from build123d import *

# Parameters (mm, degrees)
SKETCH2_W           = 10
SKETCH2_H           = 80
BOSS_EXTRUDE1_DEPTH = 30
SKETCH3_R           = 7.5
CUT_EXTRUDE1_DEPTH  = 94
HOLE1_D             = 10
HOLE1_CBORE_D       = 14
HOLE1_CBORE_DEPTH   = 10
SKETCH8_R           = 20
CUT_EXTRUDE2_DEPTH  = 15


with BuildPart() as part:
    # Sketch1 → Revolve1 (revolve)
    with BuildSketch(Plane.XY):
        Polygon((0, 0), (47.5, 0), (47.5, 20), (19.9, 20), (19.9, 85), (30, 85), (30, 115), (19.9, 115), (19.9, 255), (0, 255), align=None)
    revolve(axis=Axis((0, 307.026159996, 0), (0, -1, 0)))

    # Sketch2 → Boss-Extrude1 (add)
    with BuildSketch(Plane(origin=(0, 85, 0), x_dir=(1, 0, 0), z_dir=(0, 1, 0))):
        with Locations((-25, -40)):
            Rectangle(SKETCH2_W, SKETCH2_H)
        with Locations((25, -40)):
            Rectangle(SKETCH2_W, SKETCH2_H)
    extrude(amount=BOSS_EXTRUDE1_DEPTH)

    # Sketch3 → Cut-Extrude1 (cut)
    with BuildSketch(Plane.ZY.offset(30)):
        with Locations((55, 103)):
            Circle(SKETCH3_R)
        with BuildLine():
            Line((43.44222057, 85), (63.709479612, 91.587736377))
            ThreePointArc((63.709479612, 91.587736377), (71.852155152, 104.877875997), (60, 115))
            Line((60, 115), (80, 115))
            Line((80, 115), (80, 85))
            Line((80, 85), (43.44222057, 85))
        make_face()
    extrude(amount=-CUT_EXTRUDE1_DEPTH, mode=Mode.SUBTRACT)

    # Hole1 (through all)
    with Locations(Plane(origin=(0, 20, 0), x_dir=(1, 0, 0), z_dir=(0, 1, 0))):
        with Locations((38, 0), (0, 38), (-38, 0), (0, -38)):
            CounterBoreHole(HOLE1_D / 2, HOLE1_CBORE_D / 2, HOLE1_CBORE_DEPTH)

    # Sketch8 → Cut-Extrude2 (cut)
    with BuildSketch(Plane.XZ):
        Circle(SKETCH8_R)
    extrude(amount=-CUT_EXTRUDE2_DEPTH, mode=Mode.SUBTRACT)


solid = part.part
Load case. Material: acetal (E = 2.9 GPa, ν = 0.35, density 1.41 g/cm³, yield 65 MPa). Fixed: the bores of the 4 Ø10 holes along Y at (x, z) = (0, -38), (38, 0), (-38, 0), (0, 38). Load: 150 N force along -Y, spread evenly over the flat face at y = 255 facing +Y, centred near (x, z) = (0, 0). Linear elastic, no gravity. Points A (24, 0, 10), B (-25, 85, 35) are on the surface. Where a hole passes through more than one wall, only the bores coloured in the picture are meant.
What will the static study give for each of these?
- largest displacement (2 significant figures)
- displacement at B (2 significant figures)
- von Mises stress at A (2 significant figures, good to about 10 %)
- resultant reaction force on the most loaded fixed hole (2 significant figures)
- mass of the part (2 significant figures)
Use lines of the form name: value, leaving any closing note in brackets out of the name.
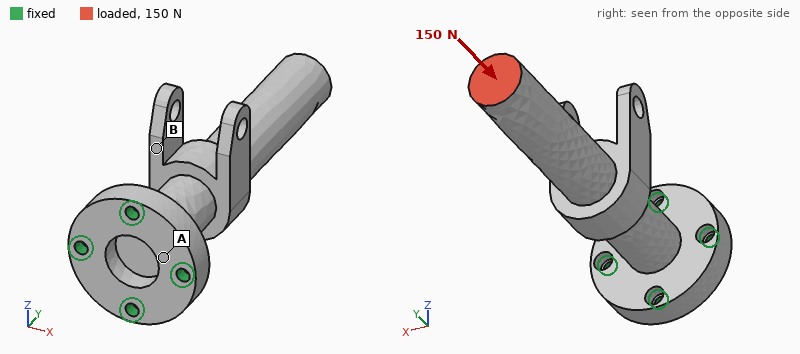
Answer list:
largest displacement: 12 µm
displacement at B: 6.1 µm
von Mises stress at A: 0.087 MPa
resultant reaction force on the most loaded fixed hole: 47 N
mass of the part: 680 g
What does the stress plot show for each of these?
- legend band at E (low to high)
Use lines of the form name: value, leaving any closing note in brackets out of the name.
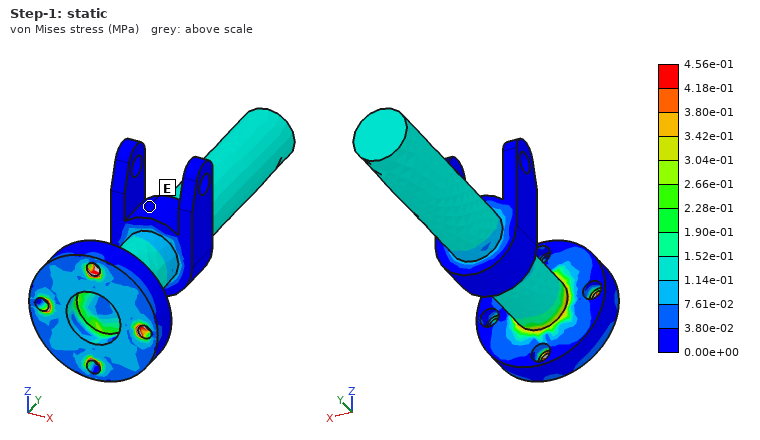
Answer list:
legend band at E: 0.00e+00 to 3.80e-02 MPa
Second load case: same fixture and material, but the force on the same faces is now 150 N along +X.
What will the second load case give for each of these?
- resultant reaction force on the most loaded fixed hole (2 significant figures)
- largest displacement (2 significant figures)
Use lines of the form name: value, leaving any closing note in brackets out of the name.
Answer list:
resultant reaction force on the most loaded fixed hole: 590 N
largest displacement: 2.3 mm
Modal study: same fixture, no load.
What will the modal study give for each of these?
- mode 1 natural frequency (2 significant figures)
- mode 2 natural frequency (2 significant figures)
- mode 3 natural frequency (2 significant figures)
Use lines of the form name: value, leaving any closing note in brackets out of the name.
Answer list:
mode 1 natural frequency: 120 Hz
mode 2 natural frequency: 120 Hz
mode 3 natural frequency: 560 Hz
